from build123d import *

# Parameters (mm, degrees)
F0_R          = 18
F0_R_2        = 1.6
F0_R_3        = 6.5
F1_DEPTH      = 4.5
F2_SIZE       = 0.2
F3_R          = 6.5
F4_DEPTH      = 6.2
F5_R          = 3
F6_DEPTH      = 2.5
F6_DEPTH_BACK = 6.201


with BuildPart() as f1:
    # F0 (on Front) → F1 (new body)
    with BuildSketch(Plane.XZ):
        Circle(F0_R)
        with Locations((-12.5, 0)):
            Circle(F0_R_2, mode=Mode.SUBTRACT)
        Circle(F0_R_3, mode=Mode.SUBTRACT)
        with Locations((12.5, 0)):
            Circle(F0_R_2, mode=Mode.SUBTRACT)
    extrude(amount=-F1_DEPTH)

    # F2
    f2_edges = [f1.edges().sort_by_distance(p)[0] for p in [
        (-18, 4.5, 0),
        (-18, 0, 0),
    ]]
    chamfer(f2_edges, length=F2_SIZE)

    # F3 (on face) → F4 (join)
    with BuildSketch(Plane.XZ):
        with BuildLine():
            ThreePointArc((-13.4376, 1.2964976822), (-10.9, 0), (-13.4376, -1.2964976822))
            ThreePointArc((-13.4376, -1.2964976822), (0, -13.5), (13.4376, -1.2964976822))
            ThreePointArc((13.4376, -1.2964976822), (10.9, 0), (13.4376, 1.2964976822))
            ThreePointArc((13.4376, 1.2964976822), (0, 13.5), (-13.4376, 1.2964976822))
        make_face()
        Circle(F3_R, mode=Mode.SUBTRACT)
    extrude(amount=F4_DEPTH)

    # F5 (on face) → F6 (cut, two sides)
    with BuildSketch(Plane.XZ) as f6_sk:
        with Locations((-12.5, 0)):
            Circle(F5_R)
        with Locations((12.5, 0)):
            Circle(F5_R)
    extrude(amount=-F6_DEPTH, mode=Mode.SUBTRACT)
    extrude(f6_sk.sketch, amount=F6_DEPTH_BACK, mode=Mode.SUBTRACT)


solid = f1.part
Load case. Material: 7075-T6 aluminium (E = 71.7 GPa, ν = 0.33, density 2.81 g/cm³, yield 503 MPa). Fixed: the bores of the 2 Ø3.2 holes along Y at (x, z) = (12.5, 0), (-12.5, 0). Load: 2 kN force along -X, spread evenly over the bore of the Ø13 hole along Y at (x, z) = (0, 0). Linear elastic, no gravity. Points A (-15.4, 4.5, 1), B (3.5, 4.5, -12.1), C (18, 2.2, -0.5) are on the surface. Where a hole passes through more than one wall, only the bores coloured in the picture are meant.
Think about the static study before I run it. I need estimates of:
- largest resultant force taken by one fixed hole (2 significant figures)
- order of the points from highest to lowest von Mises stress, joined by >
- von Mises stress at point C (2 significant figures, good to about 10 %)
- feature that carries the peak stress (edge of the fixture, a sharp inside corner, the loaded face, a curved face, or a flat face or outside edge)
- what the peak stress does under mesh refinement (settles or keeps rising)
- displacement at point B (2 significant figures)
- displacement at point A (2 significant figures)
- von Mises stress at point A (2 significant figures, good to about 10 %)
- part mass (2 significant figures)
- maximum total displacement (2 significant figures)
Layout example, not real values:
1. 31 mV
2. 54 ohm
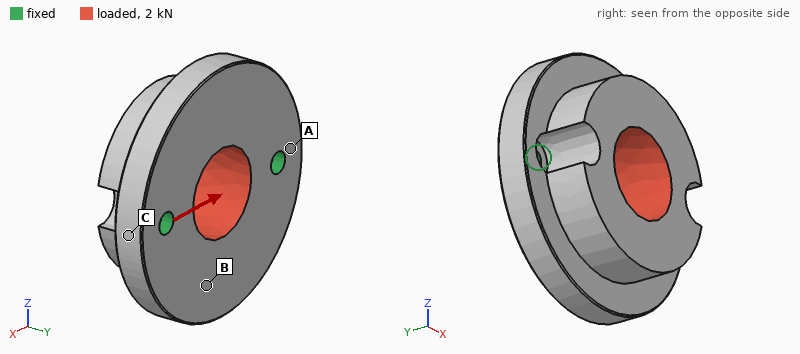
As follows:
1. 1.1 kN
2. A > C > B
3. 18 MPa
4. edge of the fixture
5. keeps rising
6. 3.9 µm
7. 1.3 µm
8. 30 MPa
9. 18 g
10. 7.1 µm
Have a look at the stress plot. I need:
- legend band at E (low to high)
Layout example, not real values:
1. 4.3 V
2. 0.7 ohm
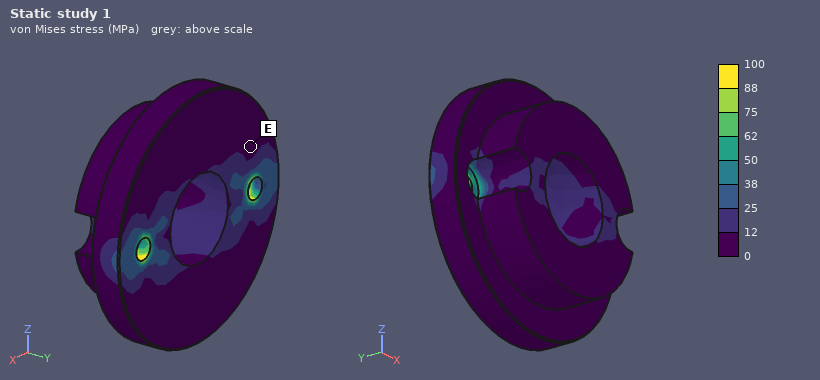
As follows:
1. 0 to 12 MPa
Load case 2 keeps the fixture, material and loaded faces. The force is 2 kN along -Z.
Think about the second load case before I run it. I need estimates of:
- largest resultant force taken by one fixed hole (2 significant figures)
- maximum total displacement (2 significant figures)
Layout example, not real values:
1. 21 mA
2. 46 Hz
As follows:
1. 1.0 kN
2. 94 µm
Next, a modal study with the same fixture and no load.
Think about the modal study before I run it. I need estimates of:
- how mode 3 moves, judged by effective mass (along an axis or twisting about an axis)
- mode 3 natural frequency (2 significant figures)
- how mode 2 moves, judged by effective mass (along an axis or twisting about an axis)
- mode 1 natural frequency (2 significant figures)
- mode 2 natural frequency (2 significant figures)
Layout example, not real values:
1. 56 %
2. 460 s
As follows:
1. twisting about Y
2. 23 kHz
3. along Y
4. 5000 Hz
5. 16 kHz
